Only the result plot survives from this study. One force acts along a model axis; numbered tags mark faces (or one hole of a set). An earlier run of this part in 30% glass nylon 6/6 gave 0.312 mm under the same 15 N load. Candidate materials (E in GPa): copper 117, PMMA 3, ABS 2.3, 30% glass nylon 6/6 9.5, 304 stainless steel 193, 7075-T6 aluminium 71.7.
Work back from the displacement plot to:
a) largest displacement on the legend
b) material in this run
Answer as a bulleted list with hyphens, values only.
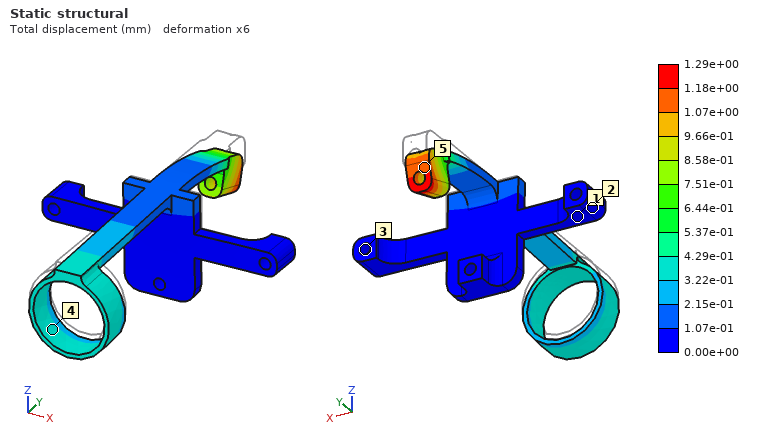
- 1.29e+00 mm
- ABS
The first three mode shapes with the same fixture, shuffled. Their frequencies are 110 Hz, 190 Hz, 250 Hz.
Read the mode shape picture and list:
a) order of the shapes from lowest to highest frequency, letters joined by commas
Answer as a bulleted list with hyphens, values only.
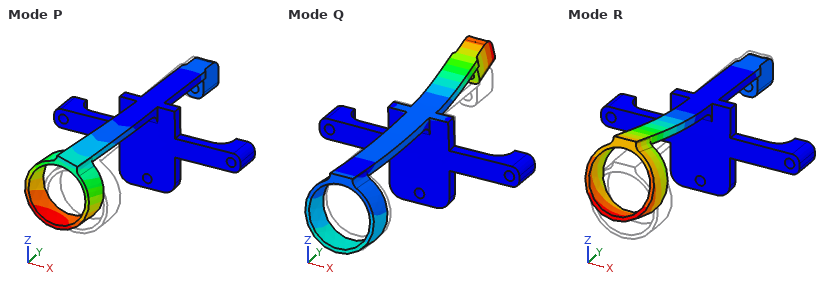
- R, P, Q
